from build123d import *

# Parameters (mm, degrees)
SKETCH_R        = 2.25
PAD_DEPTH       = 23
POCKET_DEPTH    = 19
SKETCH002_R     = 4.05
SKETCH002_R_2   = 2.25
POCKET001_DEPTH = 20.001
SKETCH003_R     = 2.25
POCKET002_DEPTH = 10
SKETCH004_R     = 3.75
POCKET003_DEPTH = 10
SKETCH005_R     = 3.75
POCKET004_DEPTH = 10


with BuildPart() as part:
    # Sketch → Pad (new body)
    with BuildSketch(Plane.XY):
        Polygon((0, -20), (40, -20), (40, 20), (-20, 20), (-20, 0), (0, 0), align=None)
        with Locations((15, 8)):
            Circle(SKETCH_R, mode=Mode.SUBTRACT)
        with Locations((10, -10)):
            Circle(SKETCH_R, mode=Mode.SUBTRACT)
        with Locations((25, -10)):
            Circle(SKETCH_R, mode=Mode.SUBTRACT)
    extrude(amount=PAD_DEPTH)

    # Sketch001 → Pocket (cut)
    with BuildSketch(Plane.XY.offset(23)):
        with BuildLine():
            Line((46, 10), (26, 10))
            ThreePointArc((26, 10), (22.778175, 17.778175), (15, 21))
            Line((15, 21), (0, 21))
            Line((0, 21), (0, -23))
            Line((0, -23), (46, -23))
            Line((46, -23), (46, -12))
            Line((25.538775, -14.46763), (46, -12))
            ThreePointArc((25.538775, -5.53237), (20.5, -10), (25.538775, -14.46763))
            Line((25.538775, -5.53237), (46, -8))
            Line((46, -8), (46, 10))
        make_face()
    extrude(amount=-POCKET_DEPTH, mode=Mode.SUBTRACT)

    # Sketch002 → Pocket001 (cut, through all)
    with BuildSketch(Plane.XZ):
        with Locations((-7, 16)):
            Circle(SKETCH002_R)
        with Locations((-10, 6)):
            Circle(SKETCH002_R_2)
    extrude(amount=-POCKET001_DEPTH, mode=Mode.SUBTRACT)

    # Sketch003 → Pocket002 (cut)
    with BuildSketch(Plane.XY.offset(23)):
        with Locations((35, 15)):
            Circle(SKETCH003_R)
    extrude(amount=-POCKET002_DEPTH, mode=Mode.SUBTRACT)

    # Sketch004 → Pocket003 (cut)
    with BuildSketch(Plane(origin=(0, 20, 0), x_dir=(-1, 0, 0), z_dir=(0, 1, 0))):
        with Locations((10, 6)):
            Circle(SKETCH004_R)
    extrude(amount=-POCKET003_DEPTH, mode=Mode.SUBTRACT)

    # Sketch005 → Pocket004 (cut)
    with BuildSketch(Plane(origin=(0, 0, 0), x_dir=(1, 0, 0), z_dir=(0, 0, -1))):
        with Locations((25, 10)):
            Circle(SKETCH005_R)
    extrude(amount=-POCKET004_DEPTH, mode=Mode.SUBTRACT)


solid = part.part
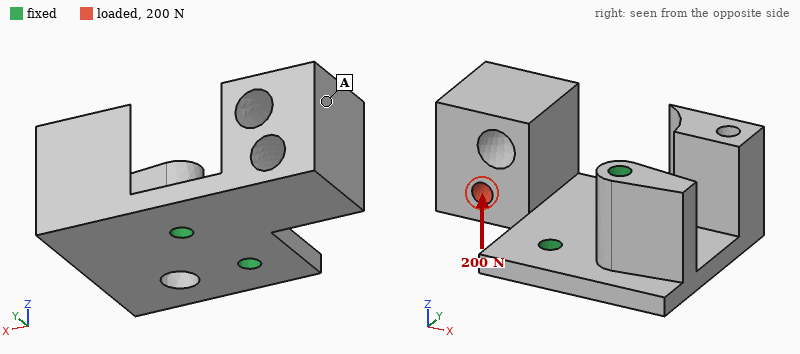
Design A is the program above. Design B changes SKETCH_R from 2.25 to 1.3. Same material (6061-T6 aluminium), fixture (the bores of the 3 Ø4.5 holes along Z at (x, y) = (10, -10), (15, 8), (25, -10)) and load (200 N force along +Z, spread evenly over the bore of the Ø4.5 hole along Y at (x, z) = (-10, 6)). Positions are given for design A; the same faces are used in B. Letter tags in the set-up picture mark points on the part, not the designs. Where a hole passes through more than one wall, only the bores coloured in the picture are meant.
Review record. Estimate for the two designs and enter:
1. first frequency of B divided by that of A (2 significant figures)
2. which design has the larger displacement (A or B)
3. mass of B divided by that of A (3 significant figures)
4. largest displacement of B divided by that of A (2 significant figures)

0.94
B
1.01
1.1
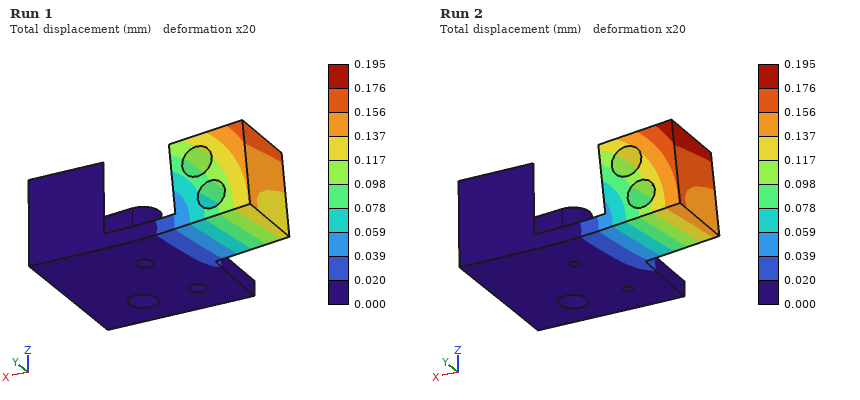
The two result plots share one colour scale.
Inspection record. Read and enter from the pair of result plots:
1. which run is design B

Run 2
